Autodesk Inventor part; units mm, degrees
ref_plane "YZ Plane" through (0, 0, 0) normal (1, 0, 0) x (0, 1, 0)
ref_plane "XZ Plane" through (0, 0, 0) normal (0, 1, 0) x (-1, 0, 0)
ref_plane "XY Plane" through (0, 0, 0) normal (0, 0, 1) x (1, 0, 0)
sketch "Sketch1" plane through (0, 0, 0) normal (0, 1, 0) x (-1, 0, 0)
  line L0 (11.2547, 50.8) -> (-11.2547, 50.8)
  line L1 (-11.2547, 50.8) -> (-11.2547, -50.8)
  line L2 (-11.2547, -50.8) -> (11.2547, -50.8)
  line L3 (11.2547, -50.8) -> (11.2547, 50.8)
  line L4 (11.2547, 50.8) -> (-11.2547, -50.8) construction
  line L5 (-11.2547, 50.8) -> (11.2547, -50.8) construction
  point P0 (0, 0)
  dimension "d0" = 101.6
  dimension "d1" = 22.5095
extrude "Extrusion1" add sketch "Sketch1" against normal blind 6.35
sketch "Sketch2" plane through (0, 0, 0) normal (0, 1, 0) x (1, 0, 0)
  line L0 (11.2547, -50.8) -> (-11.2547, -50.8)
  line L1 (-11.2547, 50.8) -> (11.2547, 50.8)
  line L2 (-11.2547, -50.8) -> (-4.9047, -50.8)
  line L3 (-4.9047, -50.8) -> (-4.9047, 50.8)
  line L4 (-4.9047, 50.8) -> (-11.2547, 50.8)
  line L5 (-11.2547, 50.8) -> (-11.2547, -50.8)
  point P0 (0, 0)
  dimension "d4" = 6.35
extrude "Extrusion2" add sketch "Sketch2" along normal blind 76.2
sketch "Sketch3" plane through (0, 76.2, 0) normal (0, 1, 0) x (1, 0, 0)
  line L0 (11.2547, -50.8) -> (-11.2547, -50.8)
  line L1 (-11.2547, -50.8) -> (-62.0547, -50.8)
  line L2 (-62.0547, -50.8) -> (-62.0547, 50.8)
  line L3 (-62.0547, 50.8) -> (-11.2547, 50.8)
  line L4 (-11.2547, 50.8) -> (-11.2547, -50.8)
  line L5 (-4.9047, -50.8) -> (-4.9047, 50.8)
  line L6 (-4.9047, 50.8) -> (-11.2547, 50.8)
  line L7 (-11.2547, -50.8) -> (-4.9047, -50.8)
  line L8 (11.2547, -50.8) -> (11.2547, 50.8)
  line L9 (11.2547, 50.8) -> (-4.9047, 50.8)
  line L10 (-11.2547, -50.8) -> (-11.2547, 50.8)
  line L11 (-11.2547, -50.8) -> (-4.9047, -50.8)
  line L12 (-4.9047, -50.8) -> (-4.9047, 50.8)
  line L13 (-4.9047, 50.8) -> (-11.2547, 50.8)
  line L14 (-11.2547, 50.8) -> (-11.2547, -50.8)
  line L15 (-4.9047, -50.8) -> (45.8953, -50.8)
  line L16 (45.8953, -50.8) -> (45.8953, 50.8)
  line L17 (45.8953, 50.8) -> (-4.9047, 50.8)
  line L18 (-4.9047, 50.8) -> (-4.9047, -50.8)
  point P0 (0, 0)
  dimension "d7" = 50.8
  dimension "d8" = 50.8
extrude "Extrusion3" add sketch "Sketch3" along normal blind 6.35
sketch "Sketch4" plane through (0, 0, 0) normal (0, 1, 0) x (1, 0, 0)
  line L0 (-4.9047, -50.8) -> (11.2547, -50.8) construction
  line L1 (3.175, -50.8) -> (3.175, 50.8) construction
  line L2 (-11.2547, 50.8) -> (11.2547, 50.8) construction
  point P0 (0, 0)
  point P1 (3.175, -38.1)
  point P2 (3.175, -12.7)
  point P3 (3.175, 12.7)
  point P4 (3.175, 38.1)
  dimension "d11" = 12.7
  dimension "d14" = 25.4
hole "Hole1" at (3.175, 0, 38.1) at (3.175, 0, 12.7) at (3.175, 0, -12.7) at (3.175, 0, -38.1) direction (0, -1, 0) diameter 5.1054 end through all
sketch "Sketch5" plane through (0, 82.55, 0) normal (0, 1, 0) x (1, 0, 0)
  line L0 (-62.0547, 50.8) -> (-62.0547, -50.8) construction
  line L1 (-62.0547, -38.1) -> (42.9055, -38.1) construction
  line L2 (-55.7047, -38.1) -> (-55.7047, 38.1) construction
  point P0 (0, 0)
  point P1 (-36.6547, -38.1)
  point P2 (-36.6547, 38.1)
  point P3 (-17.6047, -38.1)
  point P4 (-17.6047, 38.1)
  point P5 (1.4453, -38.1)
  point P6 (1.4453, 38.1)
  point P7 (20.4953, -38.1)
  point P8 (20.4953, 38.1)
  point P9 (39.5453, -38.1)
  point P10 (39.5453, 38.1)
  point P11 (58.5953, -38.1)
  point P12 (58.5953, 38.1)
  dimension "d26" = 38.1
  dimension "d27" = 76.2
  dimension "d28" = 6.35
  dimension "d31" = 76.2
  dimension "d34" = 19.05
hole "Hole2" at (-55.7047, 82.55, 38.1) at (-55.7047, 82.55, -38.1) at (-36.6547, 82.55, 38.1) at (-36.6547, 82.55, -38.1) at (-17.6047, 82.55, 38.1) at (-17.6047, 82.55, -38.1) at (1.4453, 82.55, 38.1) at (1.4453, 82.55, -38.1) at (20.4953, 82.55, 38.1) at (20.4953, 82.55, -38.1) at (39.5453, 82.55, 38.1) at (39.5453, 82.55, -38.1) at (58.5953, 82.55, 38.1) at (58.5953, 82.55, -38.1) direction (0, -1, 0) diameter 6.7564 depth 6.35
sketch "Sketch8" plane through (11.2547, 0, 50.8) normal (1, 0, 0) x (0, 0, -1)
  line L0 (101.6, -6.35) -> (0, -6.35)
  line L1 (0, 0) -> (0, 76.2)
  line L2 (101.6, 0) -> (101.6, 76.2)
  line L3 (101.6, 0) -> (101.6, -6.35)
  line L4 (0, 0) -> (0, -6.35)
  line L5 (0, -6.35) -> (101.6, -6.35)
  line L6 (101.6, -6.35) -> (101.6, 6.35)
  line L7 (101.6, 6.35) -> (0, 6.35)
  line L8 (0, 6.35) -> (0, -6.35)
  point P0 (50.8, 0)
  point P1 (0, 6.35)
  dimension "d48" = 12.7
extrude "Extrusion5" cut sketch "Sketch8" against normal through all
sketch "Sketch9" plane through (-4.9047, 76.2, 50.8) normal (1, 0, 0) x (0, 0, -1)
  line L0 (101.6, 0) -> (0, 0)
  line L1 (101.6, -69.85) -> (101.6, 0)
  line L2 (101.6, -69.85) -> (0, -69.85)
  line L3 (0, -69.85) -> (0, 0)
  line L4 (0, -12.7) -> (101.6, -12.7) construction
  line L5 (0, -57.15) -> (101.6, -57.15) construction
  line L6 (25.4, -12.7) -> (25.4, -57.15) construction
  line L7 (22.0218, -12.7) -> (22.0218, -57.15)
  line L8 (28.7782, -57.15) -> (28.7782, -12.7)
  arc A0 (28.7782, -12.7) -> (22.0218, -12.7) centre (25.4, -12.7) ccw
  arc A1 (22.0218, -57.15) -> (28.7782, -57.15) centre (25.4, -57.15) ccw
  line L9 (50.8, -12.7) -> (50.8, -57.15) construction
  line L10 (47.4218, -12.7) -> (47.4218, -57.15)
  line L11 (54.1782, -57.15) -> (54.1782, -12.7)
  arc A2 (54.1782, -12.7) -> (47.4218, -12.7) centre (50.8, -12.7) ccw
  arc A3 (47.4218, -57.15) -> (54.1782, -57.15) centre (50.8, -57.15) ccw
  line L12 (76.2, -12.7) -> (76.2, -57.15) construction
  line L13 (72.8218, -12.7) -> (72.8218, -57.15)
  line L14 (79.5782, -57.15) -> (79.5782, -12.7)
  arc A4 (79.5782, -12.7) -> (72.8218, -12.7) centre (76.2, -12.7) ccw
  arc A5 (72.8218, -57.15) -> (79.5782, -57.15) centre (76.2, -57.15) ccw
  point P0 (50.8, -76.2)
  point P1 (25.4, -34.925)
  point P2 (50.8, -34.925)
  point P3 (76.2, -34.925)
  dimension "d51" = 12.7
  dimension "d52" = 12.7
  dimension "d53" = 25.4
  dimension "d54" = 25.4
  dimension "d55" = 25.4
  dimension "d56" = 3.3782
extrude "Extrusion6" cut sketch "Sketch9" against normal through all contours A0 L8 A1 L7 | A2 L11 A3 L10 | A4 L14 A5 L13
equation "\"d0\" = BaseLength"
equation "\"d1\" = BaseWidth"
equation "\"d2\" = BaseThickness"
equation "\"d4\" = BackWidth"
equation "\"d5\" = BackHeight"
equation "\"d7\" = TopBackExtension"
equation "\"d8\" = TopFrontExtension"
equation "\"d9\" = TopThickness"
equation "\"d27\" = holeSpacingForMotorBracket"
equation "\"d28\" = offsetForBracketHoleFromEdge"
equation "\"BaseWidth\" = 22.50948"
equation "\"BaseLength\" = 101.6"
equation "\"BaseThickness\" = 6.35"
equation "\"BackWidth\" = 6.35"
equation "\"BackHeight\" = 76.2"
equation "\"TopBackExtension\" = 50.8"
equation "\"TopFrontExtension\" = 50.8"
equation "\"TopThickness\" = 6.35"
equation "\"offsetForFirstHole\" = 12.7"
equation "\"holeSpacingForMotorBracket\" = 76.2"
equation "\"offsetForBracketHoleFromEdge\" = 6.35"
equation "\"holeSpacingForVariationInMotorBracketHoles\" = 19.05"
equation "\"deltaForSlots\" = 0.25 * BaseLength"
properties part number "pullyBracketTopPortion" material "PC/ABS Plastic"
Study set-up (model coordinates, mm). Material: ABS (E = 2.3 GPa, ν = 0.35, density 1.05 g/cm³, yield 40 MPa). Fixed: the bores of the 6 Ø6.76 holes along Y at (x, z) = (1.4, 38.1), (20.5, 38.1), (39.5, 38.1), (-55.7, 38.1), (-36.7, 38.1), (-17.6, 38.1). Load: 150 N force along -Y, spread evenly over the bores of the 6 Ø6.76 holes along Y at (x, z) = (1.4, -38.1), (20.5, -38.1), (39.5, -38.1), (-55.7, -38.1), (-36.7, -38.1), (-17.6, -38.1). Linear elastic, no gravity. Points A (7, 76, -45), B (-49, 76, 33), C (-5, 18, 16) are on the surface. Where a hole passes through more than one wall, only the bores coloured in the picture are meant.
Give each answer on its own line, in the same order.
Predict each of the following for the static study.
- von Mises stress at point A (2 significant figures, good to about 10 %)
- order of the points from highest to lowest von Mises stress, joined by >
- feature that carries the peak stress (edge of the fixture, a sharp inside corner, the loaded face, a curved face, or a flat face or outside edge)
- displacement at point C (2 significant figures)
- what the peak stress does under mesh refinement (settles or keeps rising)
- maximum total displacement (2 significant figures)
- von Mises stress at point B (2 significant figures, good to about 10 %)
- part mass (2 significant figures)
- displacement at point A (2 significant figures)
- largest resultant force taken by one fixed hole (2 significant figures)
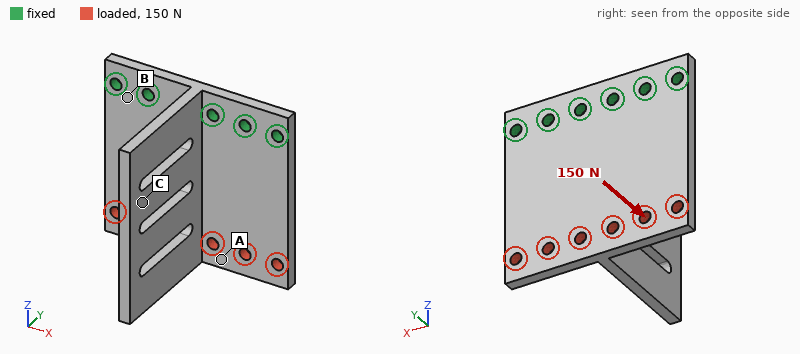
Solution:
2.4 MPa
B > A > C
edge of the fixture
0.92 mm
keeps rising
1.7 mm
5.0 MPa
110 g
1.3 mm
55 N
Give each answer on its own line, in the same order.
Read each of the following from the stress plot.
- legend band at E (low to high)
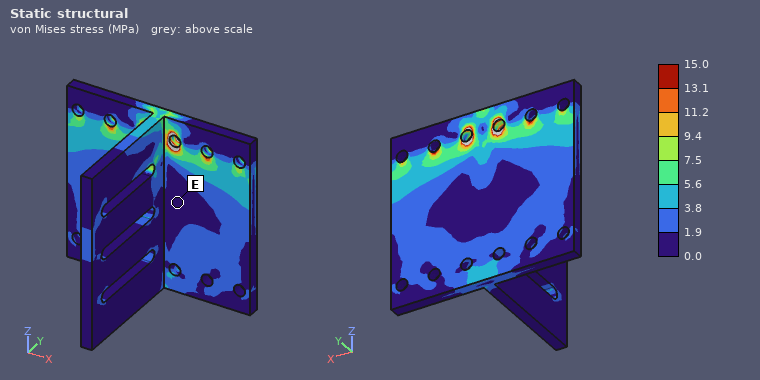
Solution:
0.0 to 1.9 MPa
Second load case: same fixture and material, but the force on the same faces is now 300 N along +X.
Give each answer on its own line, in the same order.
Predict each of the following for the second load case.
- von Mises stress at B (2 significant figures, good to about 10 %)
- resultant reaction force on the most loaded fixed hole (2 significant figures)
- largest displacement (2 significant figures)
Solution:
1.3 MPa
180 N
91 µm
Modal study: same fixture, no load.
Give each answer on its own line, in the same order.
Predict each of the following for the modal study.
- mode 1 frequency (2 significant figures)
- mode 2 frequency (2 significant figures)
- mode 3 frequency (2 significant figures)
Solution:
240 Hz
250 Hz
440 Hz
